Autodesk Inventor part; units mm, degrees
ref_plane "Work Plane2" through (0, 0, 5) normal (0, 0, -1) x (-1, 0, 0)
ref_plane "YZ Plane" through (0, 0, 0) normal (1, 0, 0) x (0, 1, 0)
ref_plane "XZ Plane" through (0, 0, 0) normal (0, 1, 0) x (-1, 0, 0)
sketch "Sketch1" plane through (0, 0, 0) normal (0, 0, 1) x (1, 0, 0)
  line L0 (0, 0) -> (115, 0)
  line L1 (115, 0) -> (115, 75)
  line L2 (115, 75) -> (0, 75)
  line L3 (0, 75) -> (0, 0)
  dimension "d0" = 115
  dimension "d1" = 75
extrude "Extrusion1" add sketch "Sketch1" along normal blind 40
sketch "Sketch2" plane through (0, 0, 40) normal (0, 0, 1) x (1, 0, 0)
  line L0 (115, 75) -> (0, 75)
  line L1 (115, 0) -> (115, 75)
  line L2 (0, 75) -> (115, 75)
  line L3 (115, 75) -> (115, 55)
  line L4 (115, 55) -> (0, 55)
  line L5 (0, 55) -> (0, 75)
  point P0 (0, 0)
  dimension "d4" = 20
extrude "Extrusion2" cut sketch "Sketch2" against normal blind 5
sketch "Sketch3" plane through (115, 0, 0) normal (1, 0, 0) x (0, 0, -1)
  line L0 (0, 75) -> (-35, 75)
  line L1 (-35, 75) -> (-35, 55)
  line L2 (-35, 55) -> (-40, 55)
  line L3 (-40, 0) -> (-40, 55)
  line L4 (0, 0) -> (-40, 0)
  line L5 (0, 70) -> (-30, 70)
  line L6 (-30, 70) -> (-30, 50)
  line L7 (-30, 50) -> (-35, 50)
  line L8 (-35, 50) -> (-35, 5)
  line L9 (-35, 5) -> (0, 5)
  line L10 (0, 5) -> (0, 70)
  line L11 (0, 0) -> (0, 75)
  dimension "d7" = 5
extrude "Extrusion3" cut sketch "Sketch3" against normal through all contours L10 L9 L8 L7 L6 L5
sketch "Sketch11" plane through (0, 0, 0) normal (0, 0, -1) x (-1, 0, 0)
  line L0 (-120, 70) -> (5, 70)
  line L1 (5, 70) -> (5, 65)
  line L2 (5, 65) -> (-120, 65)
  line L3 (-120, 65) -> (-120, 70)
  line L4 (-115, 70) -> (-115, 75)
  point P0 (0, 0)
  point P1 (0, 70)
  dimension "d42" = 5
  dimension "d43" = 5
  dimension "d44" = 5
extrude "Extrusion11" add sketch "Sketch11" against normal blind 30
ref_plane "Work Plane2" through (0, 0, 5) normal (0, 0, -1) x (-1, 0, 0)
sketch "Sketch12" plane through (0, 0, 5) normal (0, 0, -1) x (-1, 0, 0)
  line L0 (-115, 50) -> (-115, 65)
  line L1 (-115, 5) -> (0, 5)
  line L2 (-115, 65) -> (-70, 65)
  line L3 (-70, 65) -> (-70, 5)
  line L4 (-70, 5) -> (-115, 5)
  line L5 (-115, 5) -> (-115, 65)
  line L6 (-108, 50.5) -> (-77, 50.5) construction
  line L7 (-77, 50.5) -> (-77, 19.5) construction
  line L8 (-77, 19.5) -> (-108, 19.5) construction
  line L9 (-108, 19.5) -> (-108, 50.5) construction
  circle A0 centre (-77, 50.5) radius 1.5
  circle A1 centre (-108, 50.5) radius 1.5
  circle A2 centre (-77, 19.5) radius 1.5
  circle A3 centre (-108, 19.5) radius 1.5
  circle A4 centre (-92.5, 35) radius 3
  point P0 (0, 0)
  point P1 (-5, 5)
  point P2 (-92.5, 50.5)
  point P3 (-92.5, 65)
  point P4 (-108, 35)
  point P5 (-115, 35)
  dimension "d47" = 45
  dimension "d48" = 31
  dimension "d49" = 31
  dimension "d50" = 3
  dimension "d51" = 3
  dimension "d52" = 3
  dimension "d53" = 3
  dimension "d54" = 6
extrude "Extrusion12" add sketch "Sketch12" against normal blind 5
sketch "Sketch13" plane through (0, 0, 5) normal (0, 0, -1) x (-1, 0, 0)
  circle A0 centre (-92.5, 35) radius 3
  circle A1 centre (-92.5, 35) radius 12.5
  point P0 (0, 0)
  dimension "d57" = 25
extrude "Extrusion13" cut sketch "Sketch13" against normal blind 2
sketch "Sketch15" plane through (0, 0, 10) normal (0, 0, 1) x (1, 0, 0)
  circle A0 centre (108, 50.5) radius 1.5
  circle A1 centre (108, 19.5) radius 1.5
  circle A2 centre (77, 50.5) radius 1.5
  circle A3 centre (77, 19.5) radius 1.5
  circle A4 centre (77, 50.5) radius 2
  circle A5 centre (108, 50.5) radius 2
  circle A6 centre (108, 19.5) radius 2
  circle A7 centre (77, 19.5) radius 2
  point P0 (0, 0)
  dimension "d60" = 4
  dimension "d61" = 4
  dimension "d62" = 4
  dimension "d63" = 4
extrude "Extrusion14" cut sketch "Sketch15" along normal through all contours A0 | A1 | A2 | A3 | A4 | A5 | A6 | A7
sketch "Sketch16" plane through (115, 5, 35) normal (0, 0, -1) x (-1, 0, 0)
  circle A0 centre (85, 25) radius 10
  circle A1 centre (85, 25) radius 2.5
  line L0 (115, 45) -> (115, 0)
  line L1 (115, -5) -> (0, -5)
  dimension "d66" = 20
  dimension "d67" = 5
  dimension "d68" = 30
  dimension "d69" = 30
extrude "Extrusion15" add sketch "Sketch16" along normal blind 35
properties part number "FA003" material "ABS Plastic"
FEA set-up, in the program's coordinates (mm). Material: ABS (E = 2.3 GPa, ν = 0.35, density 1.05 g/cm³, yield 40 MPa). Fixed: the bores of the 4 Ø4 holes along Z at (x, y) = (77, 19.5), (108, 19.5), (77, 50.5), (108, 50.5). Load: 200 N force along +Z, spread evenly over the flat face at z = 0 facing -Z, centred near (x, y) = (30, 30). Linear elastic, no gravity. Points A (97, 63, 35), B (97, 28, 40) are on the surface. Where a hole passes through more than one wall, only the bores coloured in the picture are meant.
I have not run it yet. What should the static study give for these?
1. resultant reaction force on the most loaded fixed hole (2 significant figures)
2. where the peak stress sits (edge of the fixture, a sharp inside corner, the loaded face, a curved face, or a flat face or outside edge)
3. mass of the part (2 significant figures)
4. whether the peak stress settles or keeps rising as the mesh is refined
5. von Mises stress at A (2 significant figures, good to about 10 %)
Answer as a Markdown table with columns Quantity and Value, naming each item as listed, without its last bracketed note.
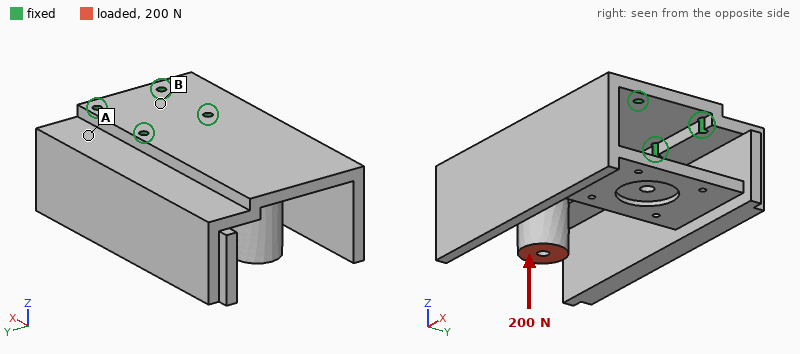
| Quantity | Value |
|---|---|
| resultant reaction force on the most loaded fixed hole | 220 N |
| where the peak stress sits | edge of the fixture |
| mass of the part | 130 g |
| whether the peak stress settles or keeps rising as the mesh is refined | keeps rising |
| von Mises stress at A | 1.8 MPa |
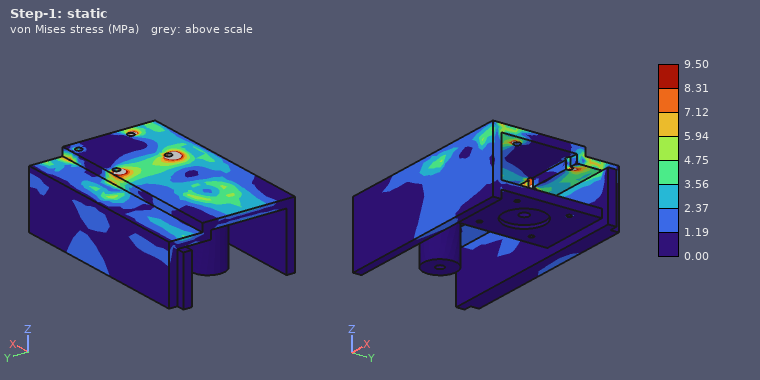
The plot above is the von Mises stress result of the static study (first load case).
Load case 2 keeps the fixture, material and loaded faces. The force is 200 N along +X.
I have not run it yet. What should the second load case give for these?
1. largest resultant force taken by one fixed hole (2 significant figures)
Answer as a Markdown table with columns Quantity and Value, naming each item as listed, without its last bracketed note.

| Quantity | Value |
|---|---|
| largest resultant force taken by one fixed hole | 130 N |
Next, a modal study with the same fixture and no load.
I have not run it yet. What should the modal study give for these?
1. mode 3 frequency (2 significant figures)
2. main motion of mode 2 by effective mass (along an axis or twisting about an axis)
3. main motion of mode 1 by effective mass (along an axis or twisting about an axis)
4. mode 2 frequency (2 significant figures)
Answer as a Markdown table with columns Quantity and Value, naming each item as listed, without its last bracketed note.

| Quantity | Value |
|---|---|
| mode 3 frequency | 640 Hz |
| main motion of mode 2 by effective mass | along Y |
| main motion of mode 1 by effective mass | along Z |
| mode 2 frequency | 370 Hz |
